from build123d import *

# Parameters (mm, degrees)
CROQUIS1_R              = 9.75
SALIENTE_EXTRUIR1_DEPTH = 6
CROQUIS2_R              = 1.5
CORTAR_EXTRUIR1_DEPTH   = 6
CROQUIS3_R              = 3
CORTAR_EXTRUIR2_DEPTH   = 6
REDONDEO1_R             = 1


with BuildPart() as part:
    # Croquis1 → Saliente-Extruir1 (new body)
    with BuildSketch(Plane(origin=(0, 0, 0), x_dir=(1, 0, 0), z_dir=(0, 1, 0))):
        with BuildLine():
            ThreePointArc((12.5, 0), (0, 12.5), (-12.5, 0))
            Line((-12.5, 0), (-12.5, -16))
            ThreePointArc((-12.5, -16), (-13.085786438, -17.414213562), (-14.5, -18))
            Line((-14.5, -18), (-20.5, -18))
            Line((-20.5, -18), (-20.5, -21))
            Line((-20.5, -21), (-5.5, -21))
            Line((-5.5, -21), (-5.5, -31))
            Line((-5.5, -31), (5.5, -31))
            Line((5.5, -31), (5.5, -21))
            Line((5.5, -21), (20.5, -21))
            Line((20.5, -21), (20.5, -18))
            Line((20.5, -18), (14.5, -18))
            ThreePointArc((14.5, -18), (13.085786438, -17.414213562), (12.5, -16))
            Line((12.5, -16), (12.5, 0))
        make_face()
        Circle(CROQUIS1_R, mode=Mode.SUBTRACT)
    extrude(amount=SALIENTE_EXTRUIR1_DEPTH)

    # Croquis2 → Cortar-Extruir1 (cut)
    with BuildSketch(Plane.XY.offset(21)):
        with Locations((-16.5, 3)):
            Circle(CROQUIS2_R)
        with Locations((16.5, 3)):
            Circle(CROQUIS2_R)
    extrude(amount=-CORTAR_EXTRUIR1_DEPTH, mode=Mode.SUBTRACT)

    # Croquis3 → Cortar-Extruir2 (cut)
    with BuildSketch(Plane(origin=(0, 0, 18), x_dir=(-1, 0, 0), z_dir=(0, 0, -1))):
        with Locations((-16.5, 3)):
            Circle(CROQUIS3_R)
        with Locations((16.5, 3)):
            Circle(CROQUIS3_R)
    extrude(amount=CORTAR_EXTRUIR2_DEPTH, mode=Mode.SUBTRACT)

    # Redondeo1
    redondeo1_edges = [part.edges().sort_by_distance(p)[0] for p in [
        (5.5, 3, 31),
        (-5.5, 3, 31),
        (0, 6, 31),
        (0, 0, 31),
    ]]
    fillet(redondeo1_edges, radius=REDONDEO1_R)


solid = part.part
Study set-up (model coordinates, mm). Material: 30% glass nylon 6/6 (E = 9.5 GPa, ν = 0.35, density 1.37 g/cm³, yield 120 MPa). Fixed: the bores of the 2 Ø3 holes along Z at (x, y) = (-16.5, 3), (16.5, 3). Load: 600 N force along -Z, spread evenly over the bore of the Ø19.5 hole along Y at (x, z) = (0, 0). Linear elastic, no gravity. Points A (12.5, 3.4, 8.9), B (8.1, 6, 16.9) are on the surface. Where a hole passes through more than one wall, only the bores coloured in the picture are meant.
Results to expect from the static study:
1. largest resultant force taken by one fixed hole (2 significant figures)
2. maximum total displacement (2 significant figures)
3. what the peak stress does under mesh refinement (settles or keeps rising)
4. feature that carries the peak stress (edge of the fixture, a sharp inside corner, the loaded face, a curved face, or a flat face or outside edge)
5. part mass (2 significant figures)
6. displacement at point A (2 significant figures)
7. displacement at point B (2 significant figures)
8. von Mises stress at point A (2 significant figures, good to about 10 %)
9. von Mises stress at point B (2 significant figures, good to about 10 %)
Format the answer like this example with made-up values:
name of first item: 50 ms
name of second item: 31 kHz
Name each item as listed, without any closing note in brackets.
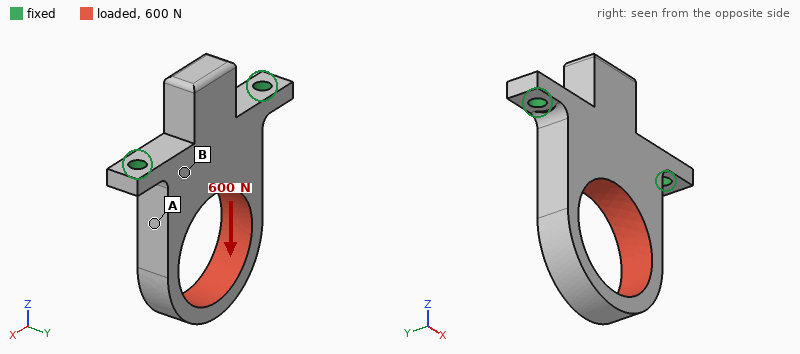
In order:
largest resultant force taken by one fixed hole: 330 N
maximum total displacement: 0.11 mm
what the peak stress does under mesh refinement: keeps rising
feature that carries the peak stress: edge of the fixture
part mass: 5.1 g
displacement at point A: 0.046 mm
displacement at point B: 0.038 mm
von Mises stress at point A: 17 MPa
von Mises stress at point B: 6.2 MPa
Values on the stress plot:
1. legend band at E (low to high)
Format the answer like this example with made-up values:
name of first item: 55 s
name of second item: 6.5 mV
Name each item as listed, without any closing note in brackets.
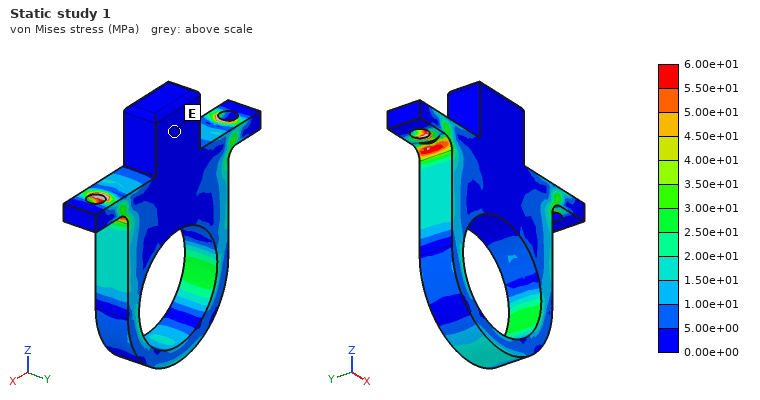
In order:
legend band at E: 0.00e+00 to 5.00e+00 MPa
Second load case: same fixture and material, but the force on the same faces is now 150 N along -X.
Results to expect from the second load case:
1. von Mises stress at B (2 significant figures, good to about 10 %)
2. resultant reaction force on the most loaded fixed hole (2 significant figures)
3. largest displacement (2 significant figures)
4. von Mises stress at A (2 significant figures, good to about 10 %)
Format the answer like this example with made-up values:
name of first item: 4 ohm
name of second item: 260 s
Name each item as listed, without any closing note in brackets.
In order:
von Mises stress at B: 3.2 MPa
resultant reaction force on the most loaded fixed hole: 130 N
largest displacement: 0.14 mm
von Mises stress at A: 12 MPa
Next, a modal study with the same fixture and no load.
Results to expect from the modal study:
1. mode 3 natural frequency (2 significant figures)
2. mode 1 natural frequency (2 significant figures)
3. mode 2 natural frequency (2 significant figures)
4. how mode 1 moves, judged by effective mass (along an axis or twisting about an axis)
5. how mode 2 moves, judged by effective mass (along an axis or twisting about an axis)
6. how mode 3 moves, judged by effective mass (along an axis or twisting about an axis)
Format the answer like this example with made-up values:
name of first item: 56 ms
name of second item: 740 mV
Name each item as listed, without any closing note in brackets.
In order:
mode 3 natural frequency: 5700 Hz
mode 1 natural frequency: 1500 Hz
mode 2 natural frequency: 4500 Hz
how mode 1 moves, judged by effective mass: along Y
how mode 2 moves, judged by effective mass: along X
how mode 3 moves, judged by effective mass: twisting about Z
